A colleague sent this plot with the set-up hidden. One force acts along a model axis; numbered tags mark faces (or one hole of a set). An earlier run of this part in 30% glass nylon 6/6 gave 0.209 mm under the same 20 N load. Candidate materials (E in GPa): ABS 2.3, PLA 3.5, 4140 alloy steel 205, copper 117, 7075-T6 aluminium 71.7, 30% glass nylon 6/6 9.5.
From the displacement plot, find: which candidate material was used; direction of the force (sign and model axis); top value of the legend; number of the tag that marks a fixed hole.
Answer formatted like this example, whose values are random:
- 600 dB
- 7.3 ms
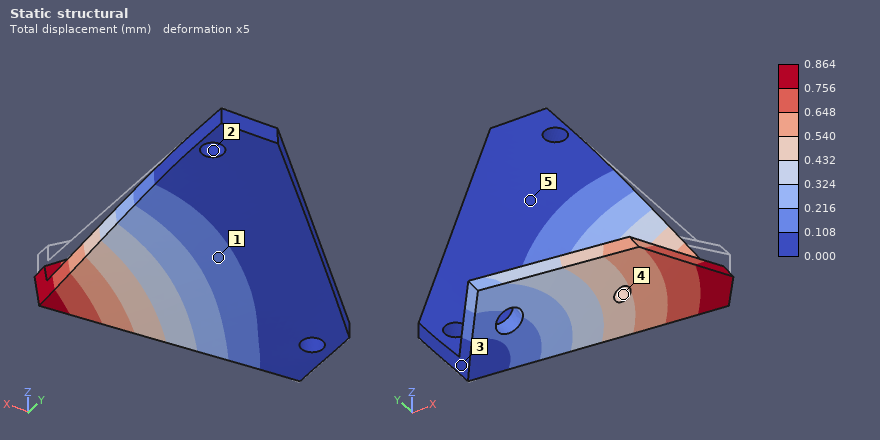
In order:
- ABS
- -Z
- 0.864 mm
- 2
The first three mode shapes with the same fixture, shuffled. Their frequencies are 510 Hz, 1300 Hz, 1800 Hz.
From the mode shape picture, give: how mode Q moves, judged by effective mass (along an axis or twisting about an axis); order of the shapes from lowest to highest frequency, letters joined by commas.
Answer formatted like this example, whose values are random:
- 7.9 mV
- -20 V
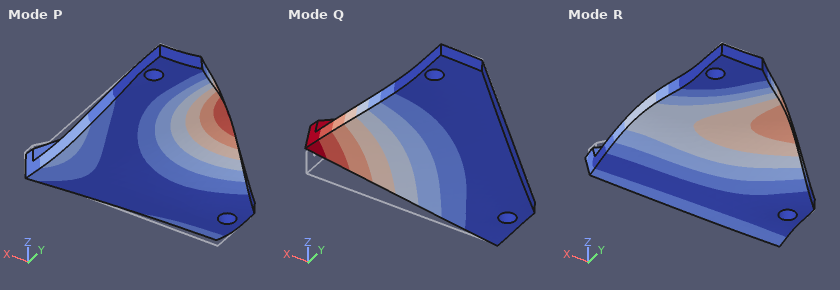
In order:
- along Z
- Q, R, P
